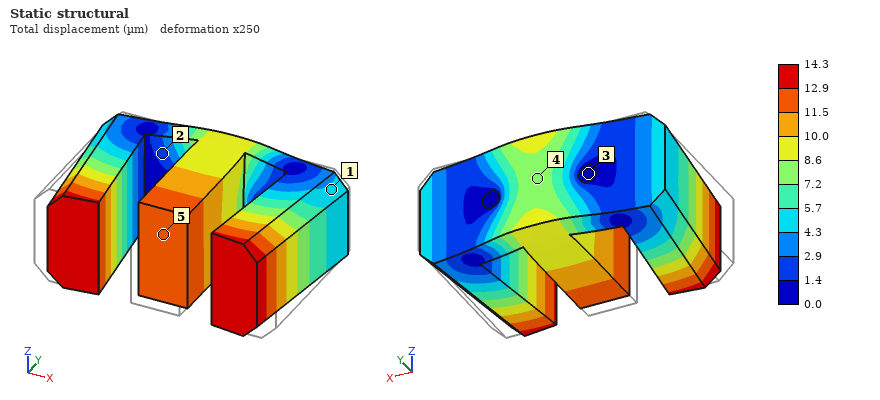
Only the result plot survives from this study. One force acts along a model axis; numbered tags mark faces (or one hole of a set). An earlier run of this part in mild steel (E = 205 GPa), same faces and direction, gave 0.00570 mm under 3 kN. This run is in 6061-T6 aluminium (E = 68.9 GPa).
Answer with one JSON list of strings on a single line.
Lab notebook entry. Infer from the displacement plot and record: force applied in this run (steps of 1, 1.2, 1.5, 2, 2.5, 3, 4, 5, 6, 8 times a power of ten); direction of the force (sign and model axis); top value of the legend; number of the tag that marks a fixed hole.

["2.5 kN", "+Y", "14.3 µm", "3"]
